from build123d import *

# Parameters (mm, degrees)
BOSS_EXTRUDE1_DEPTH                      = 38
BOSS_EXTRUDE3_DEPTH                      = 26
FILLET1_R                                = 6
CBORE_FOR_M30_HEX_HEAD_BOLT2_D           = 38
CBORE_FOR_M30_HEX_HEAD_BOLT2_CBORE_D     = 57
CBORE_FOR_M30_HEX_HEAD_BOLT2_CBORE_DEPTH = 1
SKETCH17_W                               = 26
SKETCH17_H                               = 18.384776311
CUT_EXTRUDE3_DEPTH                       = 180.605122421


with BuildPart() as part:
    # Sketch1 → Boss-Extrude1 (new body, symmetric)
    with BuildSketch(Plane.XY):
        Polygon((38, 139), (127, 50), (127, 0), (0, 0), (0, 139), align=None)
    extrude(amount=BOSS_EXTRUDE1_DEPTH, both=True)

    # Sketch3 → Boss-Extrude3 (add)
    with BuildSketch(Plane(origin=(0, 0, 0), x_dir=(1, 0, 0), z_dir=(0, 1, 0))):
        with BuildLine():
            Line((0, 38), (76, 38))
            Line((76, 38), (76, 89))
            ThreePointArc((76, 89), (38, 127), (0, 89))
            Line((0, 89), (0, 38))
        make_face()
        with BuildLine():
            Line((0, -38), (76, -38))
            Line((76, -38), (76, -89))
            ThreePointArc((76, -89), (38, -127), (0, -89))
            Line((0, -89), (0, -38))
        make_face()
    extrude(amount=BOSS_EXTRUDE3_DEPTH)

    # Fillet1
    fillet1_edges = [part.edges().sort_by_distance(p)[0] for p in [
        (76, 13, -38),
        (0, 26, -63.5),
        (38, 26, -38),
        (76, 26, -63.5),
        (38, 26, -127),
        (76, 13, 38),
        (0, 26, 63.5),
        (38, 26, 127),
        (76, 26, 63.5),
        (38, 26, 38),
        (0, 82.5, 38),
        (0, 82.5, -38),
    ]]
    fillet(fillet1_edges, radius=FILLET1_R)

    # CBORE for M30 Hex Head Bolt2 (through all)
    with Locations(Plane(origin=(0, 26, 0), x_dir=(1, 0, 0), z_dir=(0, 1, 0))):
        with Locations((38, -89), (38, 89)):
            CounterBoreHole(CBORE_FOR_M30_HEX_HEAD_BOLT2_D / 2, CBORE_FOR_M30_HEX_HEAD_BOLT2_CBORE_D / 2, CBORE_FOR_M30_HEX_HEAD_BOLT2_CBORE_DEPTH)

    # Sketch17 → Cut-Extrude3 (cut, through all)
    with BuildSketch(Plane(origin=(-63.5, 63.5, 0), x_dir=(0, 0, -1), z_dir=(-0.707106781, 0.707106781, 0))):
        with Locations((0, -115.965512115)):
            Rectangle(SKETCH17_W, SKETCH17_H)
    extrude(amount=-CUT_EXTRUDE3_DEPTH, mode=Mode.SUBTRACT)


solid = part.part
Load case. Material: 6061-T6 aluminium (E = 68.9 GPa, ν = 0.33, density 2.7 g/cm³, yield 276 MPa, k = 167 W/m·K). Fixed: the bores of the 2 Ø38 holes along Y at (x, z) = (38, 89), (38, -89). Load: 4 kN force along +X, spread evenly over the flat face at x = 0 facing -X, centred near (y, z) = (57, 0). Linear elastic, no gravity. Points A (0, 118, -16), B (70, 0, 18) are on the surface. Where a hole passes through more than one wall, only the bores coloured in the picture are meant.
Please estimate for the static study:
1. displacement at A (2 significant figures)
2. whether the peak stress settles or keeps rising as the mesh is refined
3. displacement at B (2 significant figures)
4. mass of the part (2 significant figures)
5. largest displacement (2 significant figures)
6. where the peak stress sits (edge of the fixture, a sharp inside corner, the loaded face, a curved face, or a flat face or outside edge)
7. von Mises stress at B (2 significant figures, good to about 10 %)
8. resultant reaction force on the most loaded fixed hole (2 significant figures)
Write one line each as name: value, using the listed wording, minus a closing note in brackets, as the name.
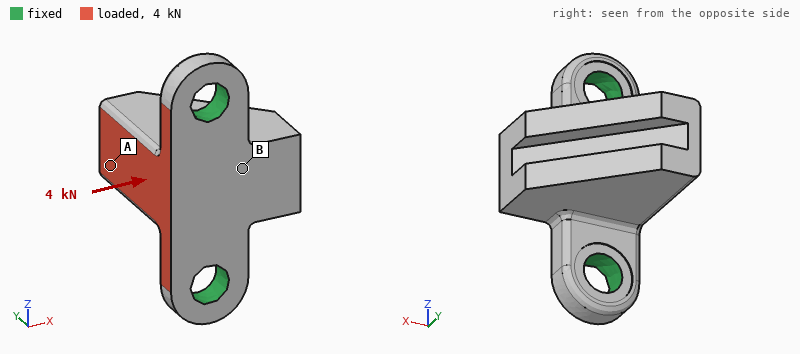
displacement at A: 41 µm
whether the peak stress settles or keeps rising as the mesh is refined: keeps rising
displacement at B: 10 µm
mass of the part: 3.3 kg
largest displacement: 48 µm
where the peak stress sits: edge of the fixture
von Mises stress at B: 3.1 MPa
resultant reaction force on the most loaded fixed hole: 2.0 kN
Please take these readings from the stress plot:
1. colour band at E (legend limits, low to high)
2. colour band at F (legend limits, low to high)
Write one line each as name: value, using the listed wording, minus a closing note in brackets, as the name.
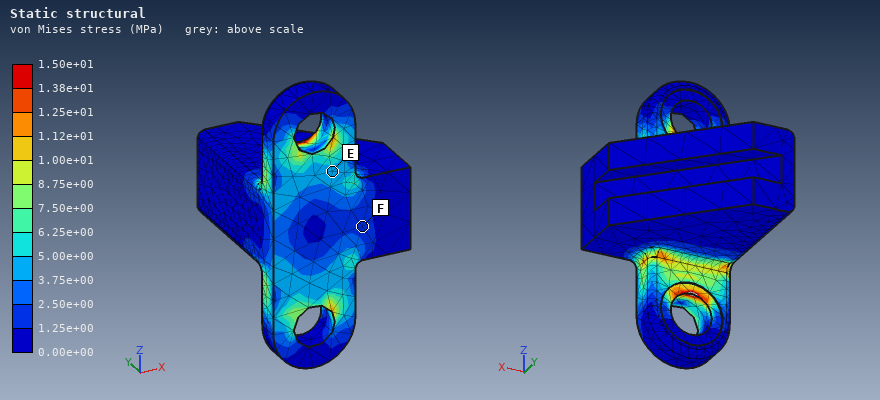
colour band at E: 3.75e+00 to 5.00e+00 MPa
colour band at F: 1.25e+00 to 2.50e+00 MPa
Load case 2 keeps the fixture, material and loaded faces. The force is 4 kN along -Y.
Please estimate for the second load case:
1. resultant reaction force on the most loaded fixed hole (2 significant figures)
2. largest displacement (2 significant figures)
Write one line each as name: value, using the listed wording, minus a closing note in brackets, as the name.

resultant reaction force on the most loaded fixed hole: 2.1 kN
largest displacement: 36 µm
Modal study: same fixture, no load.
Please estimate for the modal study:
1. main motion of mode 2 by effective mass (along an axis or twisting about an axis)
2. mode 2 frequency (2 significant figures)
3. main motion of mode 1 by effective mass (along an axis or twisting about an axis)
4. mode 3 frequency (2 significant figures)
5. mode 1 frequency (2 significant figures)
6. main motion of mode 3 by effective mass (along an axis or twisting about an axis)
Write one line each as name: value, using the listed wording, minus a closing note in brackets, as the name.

main motion of mode 2 by effective mass: along Z
mode 2 frequency: 2400 Hz
main motion of mode 1 by effective mass: along X
mode 3 frequency: 2800 Hz
mode 1 frequency: 1000 Hz
main motion of mode 3 by effective mass: along Y
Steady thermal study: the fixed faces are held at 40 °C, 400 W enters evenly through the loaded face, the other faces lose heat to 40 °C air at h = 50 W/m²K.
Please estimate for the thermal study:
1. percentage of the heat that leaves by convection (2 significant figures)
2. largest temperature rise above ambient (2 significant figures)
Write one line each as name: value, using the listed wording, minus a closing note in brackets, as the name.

percentage of the heat that leaves by convection: 19 %
largest temperature rise above ambient: 39 K
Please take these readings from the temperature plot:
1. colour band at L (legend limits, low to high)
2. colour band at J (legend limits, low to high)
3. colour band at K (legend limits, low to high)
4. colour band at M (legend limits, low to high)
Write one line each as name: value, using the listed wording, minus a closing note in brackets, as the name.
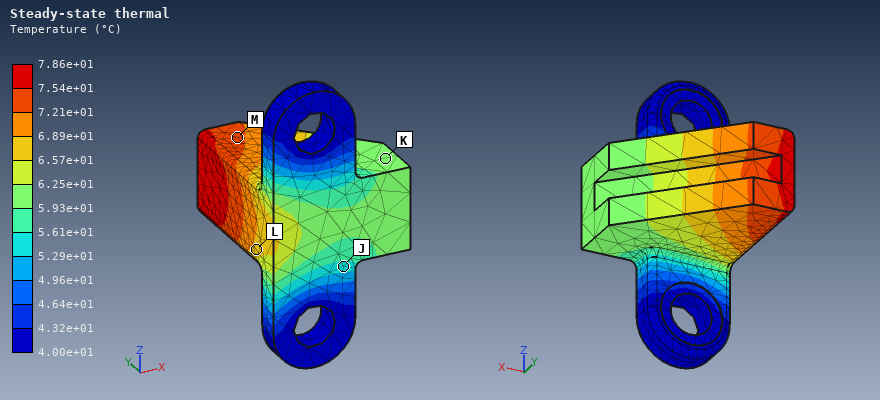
colour band at L: 6.57e+01 to 6.89e+01 °C
colour band at J: 5.29e+01 to 5.61e+01 °C
colour band at K: 5.93e+01 to 6.25e+01 °C
colour band at M: 7.21e+01 to 7.54e+01 °C
